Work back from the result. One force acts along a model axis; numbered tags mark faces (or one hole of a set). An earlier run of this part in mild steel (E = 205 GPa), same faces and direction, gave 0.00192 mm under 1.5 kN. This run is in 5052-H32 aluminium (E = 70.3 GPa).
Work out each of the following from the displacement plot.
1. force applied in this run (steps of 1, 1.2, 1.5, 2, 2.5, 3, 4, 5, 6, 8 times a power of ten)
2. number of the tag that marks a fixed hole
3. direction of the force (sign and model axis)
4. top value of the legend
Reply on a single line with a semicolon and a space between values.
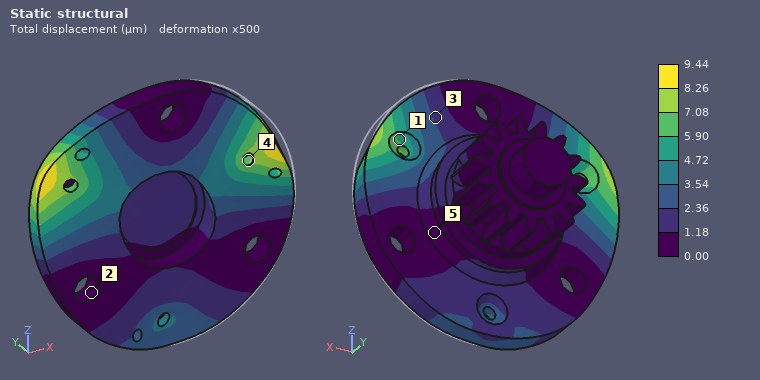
2.5 kN; 2; -X; 9.44 µm
